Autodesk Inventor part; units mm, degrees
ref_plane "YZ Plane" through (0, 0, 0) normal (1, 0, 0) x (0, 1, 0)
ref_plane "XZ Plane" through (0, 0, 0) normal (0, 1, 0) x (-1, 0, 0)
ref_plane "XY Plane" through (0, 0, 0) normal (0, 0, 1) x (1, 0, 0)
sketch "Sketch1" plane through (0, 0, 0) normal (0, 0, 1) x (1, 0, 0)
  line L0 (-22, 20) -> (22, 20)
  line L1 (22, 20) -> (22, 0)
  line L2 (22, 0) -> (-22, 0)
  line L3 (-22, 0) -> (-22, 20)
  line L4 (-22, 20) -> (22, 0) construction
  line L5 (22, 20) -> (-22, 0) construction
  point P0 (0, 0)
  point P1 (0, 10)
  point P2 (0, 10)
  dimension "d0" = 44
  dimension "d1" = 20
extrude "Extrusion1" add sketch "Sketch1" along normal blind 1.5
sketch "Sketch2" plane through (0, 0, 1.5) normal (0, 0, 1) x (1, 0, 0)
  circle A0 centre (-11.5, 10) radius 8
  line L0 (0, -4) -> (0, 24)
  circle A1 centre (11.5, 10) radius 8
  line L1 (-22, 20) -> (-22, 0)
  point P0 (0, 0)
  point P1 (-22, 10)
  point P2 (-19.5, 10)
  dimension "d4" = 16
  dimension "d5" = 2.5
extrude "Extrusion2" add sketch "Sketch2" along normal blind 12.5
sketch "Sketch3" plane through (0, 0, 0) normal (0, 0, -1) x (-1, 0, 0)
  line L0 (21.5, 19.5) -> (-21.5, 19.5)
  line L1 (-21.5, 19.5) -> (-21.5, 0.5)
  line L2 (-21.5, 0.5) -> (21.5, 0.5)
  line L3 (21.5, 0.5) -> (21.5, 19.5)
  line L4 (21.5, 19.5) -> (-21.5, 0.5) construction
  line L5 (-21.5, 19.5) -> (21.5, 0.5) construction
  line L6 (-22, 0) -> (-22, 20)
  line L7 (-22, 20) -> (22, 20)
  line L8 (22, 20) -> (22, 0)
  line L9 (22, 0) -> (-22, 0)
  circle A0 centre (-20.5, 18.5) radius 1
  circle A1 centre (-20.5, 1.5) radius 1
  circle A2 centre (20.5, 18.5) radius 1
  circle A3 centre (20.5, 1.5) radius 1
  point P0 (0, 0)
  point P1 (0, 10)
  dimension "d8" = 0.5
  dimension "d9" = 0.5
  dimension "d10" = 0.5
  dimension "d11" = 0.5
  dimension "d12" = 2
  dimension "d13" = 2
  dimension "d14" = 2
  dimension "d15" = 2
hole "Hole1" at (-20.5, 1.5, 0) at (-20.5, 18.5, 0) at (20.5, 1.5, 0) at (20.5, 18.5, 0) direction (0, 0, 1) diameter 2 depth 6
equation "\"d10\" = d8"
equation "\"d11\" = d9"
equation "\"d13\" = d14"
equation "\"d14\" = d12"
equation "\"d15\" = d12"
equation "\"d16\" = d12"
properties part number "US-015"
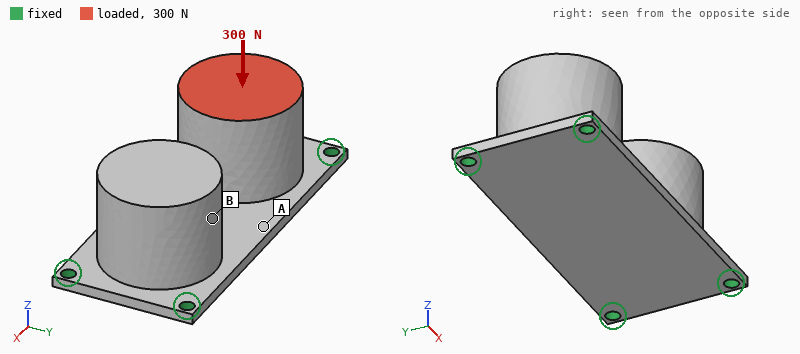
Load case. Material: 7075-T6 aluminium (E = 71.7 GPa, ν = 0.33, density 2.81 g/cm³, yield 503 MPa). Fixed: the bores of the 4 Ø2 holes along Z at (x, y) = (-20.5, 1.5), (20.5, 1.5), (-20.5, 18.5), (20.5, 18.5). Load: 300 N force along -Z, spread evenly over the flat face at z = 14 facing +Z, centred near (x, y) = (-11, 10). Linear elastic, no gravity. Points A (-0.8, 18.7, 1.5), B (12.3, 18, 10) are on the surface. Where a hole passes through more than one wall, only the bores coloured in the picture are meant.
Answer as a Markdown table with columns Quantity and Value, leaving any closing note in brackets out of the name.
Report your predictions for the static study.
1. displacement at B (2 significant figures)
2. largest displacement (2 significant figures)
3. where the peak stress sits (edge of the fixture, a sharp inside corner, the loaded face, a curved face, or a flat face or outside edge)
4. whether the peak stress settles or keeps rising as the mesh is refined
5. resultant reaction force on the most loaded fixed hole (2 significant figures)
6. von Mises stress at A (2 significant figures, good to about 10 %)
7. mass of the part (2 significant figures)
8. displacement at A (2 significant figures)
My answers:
| Quantity | Value |
|---|---|
| displacement at B | 0.068 mm |
| largest displacement | 0.14 mm |
| where the peak stress sits | edge of the fixture |
| whether the peak stress settles or keeps rising as the mesh is refined | keeps rising |
| resultant reaction force on the most loaded fixed hole | 130 N |
| von Mises stress at A | 62 MPa |
| mass of the part | 18 g |
| displacement at A | 0.10 mm |
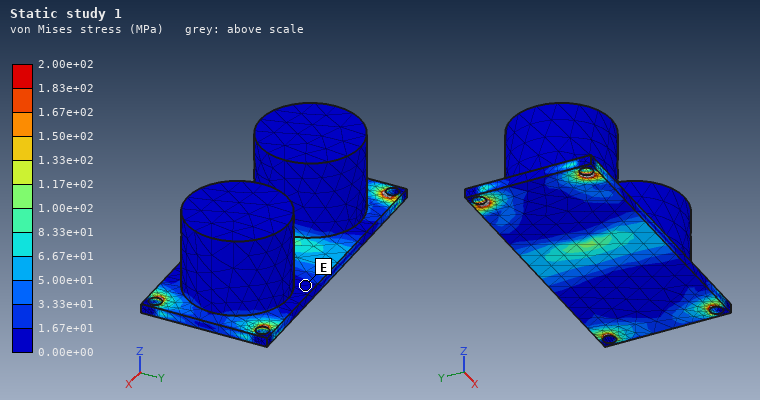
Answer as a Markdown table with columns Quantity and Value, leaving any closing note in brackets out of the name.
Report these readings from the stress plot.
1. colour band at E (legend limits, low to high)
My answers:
| Quantity | Value |
|---|---|
| colour band at E | 0.00e+00 to 1.67e+01 MPa |
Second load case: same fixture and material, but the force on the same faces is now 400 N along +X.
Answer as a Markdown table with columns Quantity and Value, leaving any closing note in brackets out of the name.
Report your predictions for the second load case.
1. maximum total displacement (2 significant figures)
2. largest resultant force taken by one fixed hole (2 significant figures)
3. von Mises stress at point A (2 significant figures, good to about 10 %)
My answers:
| Quantity | Value |
|---|---|
| maximum total displacement | 0.33 mm |
| largest resultant force taken by one fixed hole | 160 N |
| von Mises stress at point A | 150 MPa |
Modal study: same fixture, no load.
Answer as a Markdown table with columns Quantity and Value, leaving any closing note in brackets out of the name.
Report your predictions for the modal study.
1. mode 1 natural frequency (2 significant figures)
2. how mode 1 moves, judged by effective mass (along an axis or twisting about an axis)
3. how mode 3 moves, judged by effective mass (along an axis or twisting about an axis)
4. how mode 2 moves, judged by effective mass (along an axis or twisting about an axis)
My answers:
| Quantity | Value |
|---|---|
| mode 1 natural frequency | 2000 Hz |
| how mode 1 moves, judged by effective mass | along Z |
| how mode 3 moves, judged by effective mass | twisting about Z |
| how mode 2 moves, judged by effective mass | along Y |
